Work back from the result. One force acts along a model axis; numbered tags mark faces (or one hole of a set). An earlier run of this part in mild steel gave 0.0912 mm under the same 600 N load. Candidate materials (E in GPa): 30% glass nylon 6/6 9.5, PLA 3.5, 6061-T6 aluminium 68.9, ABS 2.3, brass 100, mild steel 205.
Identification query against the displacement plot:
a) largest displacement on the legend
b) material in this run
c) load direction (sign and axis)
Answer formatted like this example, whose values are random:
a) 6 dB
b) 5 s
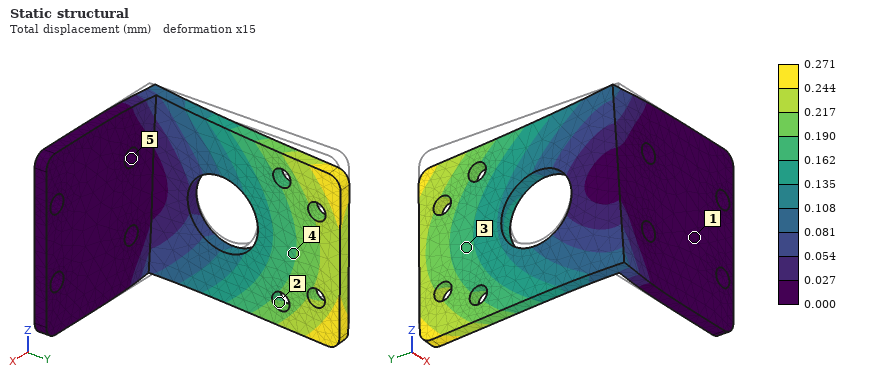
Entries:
a) 0.271 mm
b) 6061-T6 aluminium
c) -Z
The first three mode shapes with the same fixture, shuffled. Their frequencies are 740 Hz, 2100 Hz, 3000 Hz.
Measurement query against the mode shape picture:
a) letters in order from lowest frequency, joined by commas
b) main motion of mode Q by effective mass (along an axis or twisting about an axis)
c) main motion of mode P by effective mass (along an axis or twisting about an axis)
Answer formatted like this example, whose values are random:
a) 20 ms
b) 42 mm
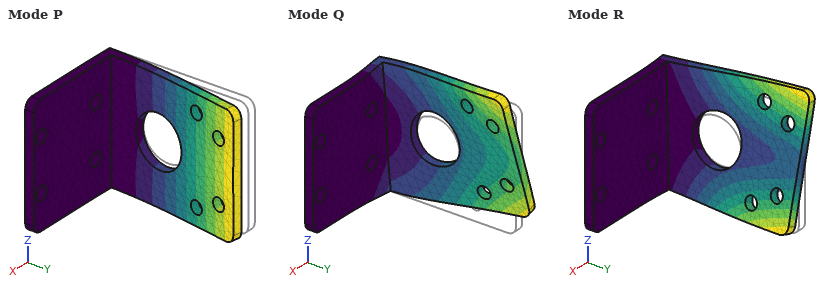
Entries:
a) P, R, Q
b) along Z
c) along X
